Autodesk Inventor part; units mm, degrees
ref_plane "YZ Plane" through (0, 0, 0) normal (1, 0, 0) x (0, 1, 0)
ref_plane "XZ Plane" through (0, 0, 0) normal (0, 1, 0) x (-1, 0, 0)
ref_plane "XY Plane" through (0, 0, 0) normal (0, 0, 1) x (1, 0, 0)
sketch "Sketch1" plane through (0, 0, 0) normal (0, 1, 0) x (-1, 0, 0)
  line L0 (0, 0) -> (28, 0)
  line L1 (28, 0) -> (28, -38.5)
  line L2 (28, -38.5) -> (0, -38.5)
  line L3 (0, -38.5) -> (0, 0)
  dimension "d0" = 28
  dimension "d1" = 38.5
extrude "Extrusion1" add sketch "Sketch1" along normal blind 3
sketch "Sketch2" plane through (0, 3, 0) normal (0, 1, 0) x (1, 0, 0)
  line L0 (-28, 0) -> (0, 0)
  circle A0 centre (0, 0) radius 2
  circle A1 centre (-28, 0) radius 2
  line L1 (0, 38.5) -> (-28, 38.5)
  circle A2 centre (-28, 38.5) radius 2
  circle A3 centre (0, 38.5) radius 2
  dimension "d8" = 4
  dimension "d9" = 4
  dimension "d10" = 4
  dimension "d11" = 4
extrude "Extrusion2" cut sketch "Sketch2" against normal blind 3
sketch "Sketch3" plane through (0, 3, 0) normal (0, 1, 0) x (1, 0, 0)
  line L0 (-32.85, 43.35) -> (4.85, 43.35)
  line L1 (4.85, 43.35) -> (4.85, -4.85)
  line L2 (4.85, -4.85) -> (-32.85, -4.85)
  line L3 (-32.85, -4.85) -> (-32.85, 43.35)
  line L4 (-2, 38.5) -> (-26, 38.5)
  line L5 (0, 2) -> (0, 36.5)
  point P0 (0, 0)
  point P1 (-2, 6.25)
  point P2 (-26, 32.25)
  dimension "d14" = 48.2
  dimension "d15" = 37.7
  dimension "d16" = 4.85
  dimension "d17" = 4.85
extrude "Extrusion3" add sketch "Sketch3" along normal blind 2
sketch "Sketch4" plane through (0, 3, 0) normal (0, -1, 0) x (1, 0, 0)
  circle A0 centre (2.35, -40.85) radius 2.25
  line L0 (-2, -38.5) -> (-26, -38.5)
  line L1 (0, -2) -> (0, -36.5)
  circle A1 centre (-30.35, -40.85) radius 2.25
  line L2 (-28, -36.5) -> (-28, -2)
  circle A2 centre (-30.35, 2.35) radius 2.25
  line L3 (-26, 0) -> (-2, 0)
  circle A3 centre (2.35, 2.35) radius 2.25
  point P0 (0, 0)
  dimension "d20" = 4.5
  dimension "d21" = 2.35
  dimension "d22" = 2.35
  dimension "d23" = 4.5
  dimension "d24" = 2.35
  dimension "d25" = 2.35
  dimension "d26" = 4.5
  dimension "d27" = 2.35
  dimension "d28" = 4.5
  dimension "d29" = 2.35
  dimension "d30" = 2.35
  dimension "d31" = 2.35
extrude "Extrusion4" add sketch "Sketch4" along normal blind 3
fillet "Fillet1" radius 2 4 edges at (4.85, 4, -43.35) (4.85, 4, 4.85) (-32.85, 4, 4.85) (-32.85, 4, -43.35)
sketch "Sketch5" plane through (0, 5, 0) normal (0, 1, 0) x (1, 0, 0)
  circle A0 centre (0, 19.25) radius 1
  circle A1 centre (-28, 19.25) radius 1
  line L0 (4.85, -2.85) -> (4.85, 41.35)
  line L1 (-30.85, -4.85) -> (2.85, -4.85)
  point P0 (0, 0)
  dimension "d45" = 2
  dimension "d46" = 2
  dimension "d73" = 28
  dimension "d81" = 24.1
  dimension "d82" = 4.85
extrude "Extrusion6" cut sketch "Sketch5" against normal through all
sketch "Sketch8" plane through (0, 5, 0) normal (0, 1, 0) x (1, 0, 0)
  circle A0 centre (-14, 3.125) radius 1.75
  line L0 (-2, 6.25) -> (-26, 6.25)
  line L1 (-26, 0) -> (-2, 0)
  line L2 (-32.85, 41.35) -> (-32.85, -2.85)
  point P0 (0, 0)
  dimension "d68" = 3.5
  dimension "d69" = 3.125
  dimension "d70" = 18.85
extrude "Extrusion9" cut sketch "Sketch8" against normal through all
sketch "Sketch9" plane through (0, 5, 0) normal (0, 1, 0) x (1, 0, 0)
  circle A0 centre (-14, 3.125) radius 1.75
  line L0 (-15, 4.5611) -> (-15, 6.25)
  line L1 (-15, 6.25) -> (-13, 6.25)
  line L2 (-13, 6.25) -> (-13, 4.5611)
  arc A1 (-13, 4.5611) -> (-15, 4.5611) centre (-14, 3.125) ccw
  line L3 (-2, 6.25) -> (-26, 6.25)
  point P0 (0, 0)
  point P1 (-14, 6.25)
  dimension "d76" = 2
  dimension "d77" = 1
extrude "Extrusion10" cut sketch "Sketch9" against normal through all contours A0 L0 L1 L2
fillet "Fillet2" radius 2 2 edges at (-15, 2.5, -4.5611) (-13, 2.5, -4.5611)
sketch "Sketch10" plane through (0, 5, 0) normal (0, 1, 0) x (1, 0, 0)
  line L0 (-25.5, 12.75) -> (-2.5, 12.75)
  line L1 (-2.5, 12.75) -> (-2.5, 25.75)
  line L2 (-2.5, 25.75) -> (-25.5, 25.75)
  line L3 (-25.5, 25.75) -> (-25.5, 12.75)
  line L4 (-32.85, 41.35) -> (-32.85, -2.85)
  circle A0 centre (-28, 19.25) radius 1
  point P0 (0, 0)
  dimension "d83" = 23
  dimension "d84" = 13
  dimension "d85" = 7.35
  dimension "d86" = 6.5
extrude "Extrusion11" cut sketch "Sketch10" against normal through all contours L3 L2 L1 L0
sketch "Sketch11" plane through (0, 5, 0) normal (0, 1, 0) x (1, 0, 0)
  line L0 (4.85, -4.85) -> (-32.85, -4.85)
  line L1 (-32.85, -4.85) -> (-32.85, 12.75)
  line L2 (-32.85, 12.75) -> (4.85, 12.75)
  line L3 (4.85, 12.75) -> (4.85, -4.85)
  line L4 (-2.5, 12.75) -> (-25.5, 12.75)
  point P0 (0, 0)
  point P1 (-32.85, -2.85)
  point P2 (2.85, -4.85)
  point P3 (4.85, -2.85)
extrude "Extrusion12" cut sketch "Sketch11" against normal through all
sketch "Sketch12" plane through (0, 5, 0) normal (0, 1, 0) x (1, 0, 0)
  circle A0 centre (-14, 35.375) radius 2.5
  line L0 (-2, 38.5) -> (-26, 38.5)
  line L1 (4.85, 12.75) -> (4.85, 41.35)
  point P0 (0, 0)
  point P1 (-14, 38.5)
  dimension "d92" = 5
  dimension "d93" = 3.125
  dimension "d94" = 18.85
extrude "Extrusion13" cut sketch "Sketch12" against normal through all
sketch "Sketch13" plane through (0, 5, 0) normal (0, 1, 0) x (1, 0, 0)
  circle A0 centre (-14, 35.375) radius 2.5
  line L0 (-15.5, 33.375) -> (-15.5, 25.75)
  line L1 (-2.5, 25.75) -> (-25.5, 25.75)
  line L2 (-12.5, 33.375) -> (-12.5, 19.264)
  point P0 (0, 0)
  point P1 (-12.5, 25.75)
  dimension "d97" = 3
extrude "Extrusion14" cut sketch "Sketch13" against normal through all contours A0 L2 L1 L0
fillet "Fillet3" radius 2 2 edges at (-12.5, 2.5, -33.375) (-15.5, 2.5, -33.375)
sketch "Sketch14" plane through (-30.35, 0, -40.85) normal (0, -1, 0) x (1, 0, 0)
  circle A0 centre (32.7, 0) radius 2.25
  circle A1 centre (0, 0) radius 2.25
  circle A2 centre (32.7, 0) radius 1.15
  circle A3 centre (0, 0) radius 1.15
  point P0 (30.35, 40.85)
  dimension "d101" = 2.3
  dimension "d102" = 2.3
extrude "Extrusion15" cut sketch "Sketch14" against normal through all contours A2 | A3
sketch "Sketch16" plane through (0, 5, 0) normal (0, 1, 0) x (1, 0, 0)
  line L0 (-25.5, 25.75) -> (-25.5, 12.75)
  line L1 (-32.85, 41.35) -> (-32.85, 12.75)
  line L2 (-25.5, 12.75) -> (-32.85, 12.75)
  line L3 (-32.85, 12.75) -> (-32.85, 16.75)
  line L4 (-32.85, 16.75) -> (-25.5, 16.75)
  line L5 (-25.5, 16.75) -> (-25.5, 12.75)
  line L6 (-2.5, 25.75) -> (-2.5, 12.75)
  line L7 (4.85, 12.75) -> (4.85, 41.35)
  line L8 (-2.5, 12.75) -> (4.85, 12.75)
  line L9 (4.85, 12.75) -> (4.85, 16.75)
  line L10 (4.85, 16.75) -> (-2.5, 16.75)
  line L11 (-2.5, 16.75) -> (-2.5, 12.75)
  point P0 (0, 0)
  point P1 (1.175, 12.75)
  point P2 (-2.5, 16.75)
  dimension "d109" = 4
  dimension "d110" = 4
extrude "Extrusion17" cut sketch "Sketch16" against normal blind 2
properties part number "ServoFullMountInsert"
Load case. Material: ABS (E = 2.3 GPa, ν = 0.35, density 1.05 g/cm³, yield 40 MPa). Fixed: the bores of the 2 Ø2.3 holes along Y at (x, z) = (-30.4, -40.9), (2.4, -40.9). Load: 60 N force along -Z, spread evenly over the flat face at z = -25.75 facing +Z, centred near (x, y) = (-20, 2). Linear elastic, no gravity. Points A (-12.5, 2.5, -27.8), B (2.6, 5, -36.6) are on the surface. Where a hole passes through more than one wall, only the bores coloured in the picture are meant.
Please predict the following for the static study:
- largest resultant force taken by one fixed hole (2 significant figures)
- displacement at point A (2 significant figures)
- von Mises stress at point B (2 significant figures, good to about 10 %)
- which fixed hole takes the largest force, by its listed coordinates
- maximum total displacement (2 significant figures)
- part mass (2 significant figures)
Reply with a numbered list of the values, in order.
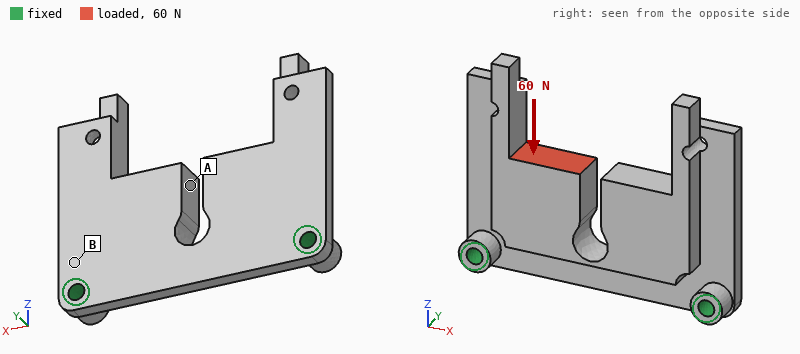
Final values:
1. 45 N
2. 0.17 mm
3. 4.4 MPa
4. (-30.4, -40.9)
5. 0.50 mm
6. 2.8 g
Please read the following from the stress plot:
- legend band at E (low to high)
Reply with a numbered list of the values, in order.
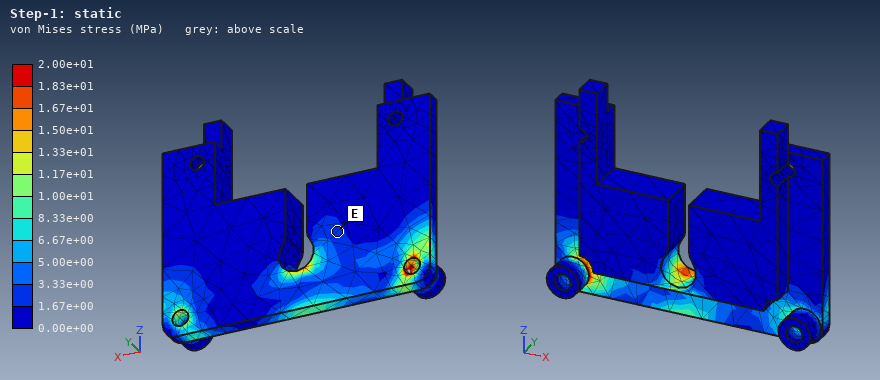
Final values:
1. 1.67e+00 to 3.33e+00 MPa
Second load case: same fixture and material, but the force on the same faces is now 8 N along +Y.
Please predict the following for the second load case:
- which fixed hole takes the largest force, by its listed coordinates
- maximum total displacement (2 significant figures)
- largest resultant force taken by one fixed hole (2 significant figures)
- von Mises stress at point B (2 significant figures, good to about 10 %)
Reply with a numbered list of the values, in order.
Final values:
1. (-30.4, -40.9)
2. 0.58 mm
3. 6.7 N
4. 2.8 MPa
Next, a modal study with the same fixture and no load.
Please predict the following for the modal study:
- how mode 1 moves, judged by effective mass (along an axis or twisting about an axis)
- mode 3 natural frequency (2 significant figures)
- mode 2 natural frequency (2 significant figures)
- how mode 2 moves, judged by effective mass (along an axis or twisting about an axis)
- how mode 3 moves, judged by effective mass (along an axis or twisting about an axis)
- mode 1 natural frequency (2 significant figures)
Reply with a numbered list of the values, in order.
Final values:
1. along Y
2. 2000 Hz
3. 1100 Hz
4. twisting about Z
5. along Z
6. 820 Hz
